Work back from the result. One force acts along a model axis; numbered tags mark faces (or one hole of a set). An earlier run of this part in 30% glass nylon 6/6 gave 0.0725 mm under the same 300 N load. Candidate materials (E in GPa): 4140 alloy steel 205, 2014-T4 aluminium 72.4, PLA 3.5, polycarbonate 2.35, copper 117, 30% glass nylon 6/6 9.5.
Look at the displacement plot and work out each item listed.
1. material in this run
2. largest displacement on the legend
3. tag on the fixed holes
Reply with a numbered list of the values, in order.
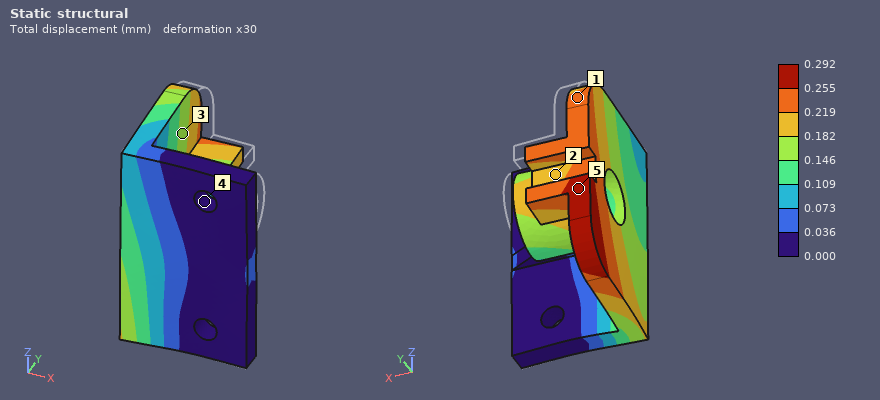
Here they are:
1. polycarbonate
2. 0.292 mm
3. 4
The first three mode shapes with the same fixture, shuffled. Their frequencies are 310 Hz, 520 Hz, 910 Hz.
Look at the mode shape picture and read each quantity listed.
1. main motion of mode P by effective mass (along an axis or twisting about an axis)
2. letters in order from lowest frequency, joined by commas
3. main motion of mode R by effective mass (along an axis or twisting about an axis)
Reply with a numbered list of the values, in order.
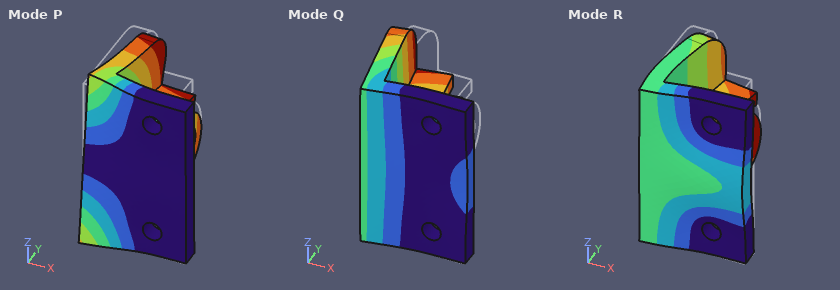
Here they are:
1. along Z
2. Q, P, R
3. along Y
